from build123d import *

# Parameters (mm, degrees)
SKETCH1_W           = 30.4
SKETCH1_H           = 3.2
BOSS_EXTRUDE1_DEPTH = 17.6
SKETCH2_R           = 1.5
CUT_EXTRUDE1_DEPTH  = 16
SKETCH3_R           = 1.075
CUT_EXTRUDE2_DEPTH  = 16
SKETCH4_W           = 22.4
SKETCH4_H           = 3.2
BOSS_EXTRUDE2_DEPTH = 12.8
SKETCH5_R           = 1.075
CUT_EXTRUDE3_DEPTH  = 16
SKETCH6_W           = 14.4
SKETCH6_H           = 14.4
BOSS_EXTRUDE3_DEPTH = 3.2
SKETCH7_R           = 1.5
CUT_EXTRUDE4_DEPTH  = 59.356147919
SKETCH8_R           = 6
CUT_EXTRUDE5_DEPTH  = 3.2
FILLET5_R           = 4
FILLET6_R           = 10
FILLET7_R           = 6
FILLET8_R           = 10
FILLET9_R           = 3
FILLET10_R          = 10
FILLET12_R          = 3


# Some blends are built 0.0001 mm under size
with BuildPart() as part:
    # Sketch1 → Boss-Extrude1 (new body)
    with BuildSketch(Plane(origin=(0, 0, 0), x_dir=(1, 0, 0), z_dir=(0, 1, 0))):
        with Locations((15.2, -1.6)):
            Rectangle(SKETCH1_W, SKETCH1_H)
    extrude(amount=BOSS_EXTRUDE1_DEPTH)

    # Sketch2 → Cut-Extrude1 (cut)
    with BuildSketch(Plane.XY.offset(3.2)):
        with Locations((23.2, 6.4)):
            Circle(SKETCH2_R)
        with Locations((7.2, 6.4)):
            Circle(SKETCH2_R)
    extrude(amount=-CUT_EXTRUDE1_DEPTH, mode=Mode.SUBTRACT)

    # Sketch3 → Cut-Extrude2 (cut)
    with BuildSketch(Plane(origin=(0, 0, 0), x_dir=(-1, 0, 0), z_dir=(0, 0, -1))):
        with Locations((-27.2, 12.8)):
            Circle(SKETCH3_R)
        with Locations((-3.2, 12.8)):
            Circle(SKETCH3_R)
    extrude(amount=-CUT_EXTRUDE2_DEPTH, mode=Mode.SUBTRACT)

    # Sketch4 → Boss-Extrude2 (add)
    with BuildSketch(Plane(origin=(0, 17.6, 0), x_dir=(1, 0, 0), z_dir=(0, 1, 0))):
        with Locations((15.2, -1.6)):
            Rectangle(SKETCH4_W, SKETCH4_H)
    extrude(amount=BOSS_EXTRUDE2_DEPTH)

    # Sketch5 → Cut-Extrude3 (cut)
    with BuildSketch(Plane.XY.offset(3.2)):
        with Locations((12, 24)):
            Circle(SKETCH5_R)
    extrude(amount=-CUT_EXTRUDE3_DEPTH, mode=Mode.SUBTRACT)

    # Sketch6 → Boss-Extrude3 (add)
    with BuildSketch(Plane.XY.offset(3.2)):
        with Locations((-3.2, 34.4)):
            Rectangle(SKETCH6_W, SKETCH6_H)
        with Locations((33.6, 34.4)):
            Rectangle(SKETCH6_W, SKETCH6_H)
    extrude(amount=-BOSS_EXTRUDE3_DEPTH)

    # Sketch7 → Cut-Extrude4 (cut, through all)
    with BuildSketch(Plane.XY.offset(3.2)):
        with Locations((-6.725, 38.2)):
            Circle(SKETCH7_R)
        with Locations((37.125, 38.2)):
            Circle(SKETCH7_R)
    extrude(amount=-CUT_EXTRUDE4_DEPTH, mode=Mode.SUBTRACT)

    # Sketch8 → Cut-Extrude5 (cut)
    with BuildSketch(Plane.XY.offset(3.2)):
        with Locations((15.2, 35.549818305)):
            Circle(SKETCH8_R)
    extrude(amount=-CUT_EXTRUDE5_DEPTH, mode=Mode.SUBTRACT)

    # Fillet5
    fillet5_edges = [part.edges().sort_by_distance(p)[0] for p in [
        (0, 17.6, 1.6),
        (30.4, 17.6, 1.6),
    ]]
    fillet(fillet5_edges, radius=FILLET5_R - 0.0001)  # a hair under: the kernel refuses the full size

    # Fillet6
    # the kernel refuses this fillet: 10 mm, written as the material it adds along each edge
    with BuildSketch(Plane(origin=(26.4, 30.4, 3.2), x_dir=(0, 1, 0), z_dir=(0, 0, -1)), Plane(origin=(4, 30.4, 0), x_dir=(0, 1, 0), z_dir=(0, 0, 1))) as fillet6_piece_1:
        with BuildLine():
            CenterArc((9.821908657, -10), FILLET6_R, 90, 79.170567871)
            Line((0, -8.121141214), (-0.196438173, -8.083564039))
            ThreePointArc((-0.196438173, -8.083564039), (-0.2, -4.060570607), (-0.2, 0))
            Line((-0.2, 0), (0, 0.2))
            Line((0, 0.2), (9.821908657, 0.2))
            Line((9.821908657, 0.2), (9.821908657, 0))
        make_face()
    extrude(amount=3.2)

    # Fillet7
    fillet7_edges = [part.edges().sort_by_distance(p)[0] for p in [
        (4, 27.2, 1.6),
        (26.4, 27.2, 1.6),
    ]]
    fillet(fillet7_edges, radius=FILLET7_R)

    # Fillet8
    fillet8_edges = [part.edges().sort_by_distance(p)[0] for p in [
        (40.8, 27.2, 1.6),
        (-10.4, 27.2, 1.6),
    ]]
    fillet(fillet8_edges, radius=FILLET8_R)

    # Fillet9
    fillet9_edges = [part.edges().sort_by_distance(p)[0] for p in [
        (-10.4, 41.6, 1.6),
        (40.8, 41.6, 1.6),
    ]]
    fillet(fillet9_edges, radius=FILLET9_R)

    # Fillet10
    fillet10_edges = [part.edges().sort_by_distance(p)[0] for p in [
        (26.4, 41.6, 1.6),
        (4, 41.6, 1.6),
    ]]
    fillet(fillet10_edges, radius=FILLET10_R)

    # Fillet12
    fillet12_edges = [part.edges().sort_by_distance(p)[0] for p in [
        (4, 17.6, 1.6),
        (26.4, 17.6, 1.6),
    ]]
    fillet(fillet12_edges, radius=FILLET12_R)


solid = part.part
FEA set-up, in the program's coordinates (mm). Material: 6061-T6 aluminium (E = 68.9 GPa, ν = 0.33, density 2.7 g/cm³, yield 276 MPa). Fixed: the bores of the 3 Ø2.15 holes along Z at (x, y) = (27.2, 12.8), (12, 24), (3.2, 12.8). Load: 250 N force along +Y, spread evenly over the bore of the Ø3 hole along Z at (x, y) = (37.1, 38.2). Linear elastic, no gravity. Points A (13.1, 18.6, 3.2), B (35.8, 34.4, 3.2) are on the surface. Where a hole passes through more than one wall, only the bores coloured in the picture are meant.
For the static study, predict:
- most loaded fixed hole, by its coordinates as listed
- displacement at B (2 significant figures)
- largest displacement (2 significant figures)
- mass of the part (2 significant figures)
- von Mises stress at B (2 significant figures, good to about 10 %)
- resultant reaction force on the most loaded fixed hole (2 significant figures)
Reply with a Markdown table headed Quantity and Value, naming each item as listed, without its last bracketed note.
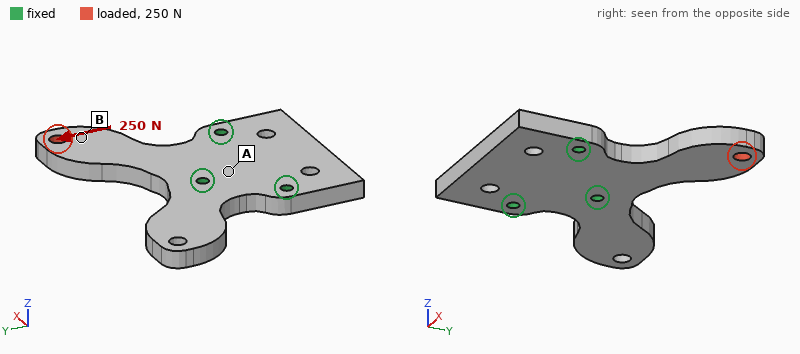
| Quantity | Value |
|---|---|
| most loaded fixed hole, by its coordinates as listed | (27.2, 12.8) |
| displacement at B | 38 µm |
| largest displacement | 58 µm |
| mass of the part | 10 g |
| von Mises stress at B | 13 MPa |
| resultant reaction force on the most loaded fixed hole | 300 N |
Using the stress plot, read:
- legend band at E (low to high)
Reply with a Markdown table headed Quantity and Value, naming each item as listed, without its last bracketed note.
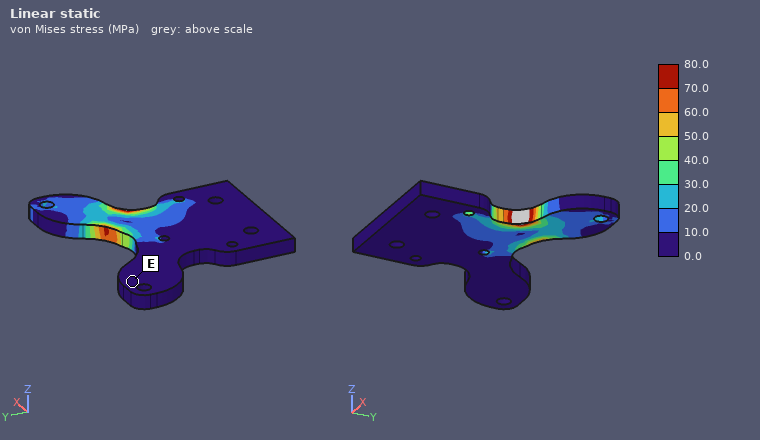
| Quantity | Value |
|---|---|
| legend band at E | 0.0 to 10.0 MPa |
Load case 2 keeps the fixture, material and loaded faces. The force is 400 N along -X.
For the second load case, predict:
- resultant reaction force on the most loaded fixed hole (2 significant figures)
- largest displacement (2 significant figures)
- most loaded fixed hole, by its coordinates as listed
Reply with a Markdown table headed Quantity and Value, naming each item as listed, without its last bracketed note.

| Quantity | Value |
|---|---|
| resultant reaction force on the most loaded fixed hole | 550 N |
| largest displacement | 74 µm |
| most loaded fixed hole, by its coordinates as listed | (12, 24) |
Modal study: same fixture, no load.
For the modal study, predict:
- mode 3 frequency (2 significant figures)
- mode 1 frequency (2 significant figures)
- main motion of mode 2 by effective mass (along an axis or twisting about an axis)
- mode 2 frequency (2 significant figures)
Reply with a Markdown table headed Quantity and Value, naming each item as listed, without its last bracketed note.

| Quantity | Value |
|---|---|
| mode 3 frequency | 11 kHz |
| mode 1 frequency | 3200 Hz |
| main motion of mode 2 by effective mass | along Z |
| mode 2 frequency | 4000 Hz |
